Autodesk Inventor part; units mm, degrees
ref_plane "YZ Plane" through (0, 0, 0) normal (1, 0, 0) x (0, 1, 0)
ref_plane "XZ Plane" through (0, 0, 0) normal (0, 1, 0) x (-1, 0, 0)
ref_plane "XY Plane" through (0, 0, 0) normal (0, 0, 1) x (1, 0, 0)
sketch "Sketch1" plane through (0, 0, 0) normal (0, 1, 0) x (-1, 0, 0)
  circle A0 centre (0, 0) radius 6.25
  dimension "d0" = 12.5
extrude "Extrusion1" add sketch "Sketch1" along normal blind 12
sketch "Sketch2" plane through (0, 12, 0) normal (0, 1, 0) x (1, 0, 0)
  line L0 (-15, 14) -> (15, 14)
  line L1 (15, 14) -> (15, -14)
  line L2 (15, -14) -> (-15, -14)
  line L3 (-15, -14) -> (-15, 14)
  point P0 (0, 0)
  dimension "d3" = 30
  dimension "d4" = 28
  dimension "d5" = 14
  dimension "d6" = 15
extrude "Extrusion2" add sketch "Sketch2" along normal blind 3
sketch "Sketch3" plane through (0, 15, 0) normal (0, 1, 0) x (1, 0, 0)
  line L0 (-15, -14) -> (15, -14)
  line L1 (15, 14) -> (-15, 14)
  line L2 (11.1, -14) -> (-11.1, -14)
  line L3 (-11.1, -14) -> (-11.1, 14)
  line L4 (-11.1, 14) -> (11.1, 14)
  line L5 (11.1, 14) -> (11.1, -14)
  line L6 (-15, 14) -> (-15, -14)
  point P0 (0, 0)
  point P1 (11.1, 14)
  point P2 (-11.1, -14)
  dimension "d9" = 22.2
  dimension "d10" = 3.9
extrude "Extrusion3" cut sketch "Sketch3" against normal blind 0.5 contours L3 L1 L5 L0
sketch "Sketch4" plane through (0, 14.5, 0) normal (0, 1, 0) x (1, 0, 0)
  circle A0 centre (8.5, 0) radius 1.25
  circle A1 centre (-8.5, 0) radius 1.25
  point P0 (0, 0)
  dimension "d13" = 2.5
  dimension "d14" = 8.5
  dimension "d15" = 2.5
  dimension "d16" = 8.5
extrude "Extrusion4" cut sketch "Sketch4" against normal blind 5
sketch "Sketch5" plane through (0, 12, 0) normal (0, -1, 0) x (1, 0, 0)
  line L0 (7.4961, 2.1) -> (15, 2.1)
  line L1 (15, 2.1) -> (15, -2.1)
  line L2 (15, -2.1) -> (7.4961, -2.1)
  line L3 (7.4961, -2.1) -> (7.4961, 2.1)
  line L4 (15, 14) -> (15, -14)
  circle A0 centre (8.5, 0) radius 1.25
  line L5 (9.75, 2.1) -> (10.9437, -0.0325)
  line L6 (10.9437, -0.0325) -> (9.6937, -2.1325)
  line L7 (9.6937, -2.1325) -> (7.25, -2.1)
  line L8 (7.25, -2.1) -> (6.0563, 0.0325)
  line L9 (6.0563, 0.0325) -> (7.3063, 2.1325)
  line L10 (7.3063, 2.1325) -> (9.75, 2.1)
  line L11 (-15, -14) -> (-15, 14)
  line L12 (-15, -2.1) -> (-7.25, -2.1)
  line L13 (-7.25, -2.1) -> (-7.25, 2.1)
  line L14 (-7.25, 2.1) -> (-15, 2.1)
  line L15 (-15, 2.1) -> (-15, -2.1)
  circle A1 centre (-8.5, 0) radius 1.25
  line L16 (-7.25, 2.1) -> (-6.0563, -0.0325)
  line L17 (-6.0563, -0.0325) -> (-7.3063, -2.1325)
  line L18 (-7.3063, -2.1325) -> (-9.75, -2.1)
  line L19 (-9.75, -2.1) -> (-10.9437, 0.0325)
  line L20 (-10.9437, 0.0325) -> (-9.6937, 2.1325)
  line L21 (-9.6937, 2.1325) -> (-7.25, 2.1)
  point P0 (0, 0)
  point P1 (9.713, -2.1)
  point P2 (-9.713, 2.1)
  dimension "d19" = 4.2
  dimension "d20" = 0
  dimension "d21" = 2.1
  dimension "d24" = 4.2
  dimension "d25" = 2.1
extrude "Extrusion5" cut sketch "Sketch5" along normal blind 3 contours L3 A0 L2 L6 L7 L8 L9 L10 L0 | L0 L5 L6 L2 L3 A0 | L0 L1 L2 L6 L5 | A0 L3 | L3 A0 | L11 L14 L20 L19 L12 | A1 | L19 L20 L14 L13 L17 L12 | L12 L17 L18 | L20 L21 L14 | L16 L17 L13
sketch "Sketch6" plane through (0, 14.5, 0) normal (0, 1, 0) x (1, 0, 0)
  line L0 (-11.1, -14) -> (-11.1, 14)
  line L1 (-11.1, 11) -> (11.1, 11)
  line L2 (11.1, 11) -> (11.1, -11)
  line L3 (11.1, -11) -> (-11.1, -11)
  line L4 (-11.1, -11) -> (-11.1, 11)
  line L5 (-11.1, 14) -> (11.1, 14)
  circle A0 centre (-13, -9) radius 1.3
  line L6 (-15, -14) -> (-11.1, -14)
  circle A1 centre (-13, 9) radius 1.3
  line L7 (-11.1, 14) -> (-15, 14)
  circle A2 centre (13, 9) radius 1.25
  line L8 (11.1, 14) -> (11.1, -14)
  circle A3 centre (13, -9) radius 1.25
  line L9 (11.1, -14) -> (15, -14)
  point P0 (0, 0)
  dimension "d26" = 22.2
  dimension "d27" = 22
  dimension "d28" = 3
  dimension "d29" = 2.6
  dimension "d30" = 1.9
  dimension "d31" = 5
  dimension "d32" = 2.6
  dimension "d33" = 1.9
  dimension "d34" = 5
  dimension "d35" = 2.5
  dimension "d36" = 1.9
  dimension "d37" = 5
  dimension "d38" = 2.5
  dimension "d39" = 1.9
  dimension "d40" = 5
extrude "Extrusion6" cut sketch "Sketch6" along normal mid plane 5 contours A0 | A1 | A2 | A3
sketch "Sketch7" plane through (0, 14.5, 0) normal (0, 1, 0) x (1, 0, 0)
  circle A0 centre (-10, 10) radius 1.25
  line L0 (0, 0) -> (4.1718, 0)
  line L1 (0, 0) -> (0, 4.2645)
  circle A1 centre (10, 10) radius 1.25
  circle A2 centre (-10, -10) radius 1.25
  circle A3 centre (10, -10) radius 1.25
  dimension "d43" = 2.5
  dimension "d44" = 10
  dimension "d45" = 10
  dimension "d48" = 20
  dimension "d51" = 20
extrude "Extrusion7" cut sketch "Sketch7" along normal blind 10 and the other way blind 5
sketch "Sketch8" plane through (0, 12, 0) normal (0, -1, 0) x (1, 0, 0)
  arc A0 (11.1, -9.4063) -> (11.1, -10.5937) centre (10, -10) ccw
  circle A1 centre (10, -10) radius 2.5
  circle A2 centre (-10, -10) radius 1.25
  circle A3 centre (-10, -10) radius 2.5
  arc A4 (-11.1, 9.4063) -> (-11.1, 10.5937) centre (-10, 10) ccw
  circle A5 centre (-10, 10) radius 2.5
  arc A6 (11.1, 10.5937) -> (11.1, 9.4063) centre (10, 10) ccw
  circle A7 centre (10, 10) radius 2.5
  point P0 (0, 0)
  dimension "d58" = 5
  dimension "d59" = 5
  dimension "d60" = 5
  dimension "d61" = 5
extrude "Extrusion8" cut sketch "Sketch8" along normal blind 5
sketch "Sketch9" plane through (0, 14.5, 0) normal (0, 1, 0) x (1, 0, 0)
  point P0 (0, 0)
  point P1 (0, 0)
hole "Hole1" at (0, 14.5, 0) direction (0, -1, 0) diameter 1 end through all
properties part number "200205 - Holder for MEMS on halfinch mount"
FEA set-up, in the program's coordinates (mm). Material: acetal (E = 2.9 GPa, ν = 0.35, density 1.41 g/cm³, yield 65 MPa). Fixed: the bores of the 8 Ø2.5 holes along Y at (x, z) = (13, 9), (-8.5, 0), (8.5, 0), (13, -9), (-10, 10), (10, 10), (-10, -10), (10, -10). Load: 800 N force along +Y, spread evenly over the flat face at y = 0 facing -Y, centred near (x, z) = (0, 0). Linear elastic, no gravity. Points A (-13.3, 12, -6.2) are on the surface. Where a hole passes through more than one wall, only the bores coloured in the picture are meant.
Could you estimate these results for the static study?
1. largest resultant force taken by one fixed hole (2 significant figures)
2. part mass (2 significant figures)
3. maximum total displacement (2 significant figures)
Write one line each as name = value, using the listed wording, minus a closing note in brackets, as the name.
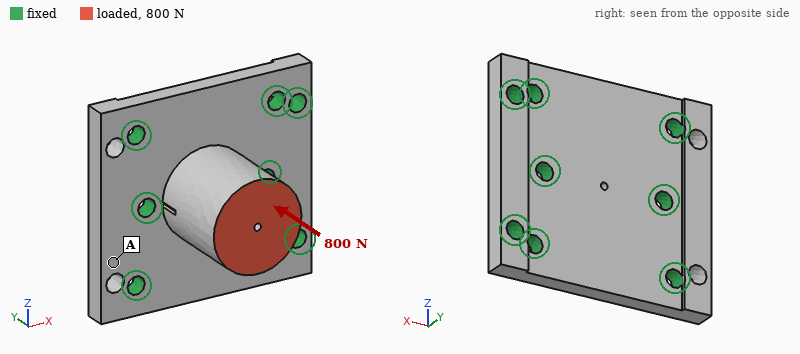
largest resultant force taken by one fixed hole = 350 N
part mass = 5.0 g
maximum total displacement = 0.11 mm
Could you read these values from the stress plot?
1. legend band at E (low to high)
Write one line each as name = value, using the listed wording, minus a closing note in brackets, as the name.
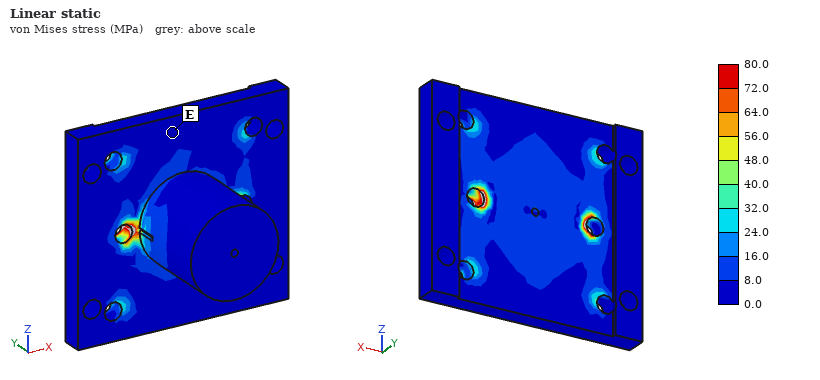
legend band at E = 0.0 to 8.0 MPa
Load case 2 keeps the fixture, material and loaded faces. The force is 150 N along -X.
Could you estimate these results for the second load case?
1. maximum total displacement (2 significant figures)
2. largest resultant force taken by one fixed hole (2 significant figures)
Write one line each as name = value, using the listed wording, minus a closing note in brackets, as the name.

maximum total displacement = 0.11 mm
largest resultant force taken by one fixed hole = 130 N
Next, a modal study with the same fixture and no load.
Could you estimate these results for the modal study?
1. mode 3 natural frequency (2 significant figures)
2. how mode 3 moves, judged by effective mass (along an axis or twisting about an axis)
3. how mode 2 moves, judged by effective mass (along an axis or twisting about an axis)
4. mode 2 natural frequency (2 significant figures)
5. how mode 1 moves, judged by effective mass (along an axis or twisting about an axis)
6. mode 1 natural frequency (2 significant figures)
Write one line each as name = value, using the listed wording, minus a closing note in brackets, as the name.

mode 3 natural frequency = 8500 Hz
how mode 3 moves, judged by effective mass = along Y
how mode 2 moves, judged by effective mass = along X
mode 2 natural frequency = 7100 Hz
how mode 1 moves, judged by effective mass = along Z
mode 1 natural frequency = 4400 Hz
